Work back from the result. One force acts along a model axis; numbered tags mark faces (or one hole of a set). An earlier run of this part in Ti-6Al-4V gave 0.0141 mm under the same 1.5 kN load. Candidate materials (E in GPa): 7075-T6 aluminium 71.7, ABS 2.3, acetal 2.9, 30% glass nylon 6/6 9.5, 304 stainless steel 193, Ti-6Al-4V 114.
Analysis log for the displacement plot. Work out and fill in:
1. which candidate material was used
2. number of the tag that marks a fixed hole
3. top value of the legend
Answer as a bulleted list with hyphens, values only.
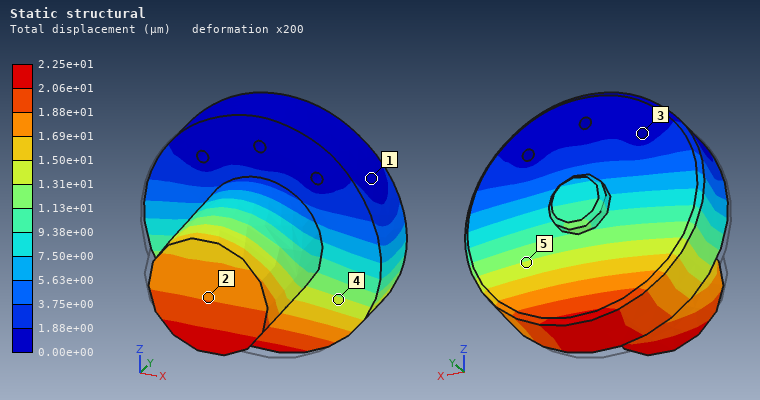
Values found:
- 7075-T6 aluminium
- 3
- 2.25e+01 µm
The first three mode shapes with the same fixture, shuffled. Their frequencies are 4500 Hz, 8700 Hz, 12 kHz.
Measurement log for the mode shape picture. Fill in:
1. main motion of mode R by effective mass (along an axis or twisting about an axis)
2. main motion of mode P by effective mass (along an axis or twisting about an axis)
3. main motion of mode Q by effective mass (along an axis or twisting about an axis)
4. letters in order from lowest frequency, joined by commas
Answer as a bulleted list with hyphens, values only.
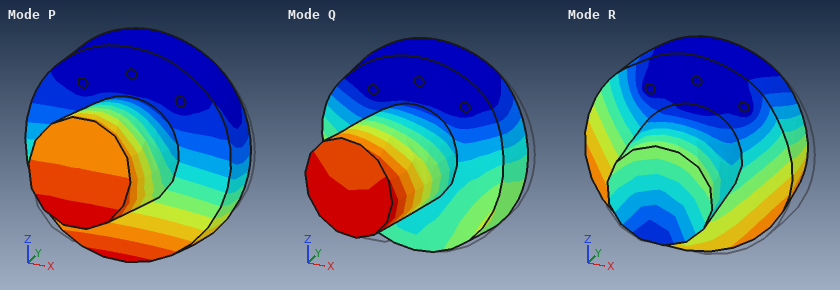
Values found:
- along X
- along Y
- along X
- P, Q, R
